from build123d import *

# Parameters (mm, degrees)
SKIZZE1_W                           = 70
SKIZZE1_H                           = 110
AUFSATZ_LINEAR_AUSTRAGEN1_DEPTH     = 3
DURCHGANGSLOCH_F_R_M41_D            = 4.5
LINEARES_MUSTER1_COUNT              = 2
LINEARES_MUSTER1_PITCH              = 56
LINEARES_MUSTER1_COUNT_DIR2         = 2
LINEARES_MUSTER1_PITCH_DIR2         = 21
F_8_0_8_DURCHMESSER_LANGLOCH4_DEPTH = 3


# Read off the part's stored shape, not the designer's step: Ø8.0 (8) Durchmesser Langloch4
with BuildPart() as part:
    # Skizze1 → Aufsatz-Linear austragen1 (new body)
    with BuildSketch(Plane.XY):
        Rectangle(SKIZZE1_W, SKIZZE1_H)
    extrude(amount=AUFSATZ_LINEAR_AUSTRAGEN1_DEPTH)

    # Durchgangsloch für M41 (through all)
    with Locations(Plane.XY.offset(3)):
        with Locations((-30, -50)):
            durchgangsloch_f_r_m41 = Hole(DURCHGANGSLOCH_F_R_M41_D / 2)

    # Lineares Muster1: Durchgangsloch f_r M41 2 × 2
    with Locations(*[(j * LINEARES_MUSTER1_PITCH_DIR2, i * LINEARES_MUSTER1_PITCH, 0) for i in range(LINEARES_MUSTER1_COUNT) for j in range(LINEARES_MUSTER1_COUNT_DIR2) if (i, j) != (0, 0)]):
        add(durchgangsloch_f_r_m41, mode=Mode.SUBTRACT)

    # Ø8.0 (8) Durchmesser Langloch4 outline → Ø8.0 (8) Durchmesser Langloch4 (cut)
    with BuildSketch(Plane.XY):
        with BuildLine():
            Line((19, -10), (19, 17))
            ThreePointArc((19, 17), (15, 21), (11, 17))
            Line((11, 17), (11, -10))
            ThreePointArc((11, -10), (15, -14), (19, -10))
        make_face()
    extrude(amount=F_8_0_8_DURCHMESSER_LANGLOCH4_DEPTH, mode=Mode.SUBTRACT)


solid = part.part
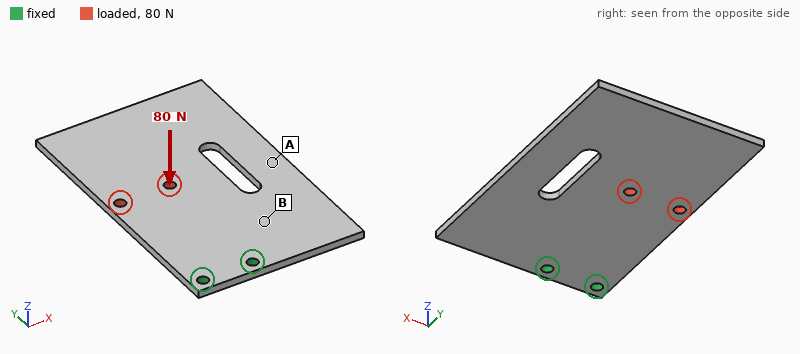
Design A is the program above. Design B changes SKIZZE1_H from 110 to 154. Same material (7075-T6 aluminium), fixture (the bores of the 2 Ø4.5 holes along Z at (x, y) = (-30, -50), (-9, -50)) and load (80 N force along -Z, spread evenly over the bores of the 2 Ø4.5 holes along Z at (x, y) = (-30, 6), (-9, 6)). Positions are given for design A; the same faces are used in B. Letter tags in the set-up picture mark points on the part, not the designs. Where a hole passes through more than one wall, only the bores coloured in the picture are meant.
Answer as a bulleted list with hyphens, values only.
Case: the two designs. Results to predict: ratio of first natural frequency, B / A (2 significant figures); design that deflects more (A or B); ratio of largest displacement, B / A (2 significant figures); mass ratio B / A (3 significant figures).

- 0.72
- B
- 1.1
- 1.42
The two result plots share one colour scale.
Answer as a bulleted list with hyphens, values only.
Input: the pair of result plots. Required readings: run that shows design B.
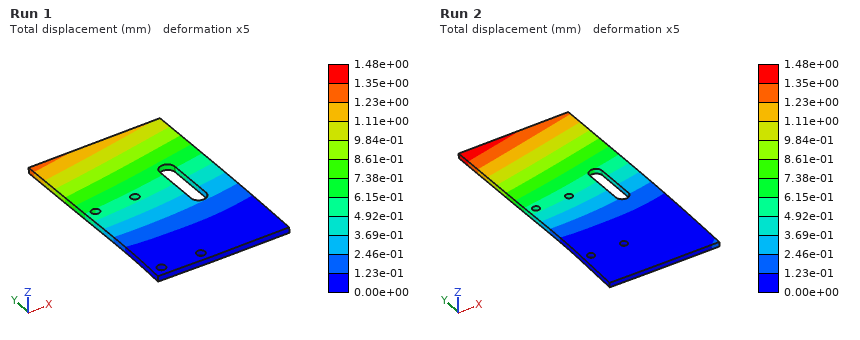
- Run 2
